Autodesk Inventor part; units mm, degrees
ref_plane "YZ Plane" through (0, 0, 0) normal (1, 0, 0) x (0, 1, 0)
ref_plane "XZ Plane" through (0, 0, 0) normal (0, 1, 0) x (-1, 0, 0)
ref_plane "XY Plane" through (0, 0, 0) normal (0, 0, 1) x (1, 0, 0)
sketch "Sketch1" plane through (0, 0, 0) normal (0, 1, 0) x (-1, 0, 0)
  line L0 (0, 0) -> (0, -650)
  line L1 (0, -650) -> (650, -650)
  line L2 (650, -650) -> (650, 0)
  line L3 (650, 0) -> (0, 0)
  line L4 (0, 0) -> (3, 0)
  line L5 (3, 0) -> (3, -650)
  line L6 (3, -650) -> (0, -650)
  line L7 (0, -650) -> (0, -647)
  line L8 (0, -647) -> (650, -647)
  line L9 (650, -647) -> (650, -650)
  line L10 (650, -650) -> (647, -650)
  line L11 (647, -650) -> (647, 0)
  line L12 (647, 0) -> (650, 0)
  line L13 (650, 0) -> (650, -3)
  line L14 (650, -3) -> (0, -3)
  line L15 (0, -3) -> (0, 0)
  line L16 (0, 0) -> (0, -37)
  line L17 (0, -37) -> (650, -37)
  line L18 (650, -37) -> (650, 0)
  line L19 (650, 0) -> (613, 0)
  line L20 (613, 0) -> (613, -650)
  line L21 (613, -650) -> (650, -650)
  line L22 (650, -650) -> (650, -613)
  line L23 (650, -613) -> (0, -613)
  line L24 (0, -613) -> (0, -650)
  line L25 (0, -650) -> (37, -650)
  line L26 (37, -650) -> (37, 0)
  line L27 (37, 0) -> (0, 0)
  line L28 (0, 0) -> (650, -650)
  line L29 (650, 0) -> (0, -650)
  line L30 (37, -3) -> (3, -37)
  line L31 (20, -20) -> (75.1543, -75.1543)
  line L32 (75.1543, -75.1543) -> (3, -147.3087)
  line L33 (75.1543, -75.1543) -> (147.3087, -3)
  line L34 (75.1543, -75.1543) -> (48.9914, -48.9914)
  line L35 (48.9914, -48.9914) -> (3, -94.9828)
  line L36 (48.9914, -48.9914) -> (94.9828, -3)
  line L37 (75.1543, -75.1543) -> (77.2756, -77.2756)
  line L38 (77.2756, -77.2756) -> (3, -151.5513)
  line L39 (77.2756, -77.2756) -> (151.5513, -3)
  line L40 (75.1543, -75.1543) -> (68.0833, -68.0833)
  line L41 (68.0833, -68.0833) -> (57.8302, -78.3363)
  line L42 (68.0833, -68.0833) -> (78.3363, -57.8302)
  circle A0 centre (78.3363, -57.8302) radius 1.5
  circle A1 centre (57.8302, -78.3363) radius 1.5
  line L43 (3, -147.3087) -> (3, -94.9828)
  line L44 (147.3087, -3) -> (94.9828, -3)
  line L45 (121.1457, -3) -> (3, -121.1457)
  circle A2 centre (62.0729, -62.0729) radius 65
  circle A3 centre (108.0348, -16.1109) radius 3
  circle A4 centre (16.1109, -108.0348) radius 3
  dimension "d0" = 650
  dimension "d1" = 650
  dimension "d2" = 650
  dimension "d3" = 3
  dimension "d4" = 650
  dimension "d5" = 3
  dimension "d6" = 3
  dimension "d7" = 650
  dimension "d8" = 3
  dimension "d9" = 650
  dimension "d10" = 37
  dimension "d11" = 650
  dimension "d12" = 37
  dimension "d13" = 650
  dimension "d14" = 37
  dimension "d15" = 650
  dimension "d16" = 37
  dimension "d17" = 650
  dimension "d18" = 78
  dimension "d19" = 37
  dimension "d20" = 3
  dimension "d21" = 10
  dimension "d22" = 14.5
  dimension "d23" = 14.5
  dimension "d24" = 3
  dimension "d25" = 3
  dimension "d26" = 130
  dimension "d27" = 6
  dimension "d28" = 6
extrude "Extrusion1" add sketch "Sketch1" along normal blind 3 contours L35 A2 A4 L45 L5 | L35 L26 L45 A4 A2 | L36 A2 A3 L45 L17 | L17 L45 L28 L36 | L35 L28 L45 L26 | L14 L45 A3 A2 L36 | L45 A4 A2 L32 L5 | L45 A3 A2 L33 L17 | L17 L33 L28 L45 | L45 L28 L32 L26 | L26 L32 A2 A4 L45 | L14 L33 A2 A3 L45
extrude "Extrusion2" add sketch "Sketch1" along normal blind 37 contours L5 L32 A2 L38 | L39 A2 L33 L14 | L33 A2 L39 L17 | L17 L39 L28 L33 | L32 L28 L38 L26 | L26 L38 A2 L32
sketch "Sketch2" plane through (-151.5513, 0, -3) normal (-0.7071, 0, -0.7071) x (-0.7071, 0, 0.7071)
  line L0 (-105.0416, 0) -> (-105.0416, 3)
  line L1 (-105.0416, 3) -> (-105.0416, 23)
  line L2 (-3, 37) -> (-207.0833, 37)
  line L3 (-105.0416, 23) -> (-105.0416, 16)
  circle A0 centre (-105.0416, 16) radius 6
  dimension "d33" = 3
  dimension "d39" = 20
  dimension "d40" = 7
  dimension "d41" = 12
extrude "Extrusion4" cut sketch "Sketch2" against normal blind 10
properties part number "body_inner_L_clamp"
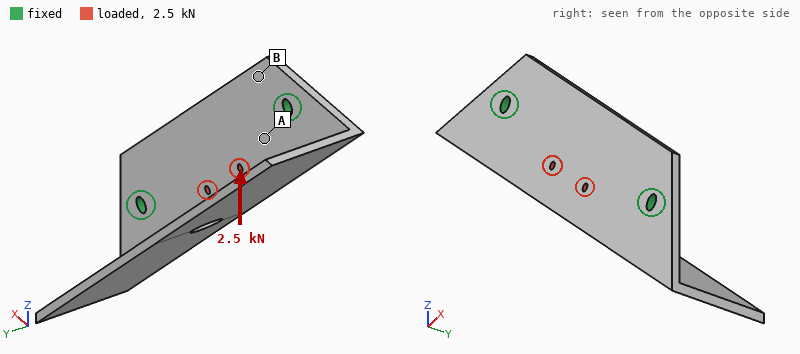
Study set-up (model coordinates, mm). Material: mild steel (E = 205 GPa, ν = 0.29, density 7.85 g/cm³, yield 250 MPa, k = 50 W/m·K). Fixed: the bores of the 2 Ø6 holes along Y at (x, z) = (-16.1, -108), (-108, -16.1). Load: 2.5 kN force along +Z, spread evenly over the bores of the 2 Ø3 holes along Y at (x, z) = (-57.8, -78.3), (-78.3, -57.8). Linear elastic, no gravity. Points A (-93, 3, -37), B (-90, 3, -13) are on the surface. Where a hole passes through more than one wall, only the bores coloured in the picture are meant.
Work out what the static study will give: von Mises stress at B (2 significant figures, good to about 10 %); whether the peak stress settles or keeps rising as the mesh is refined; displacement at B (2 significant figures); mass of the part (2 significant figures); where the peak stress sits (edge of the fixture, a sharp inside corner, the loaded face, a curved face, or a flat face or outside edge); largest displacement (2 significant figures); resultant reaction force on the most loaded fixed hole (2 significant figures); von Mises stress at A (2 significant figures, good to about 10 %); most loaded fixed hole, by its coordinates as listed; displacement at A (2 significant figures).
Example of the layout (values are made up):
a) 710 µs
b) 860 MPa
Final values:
a) 9.6 MPa
b) keeps rising
c) 7.0 µm
d) 320 g
e) edge of the fixture
f) 22 µm
g) 1.6 kN
h) 24 MPa
i) (-108, -16.1)
j) 10 µm
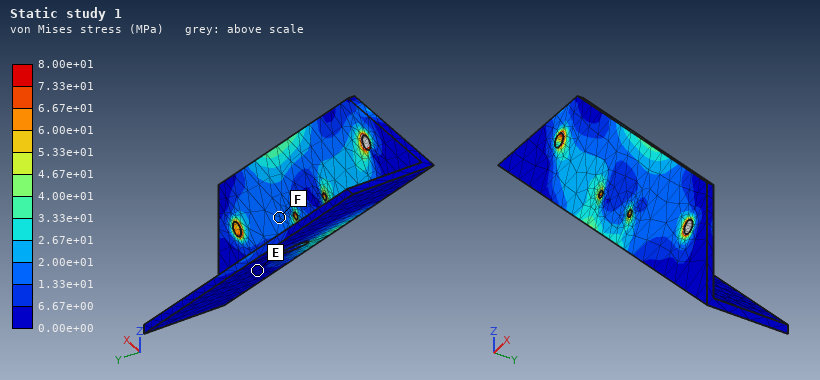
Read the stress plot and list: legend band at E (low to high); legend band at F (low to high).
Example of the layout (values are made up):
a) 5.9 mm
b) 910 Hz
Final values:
a) 0.00e+00 to 6.67e+00 MPa
b) 1.33e+01 to 2.00e+01 MPa
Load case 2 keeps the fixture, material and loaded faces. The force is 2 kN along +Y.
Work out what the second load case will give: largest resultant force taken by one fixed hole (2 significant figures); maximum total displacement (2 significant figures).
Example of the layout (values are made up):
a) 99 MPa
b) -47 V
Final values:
a) 1.1 kN
b) 0.27 mm
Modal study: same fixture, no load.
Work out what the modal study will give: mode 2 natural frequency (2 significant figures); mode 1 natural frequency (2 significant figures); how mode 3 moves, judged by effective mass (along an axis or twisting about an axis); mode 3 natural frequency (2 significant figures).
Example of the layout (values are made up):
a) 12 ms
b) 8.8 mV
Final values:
a) 1000 Hz
b) 770 Hz
c) along Y
d) 1400 Hz
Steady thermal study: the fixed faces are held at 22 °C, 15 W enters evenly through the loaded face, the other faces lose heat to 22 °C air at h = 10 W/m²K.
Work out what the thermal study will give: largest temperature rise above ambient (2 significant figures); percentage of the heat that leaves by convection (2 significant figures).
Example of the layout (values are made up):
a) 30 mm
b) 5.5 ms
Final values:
a) 53 K
b) 36 %
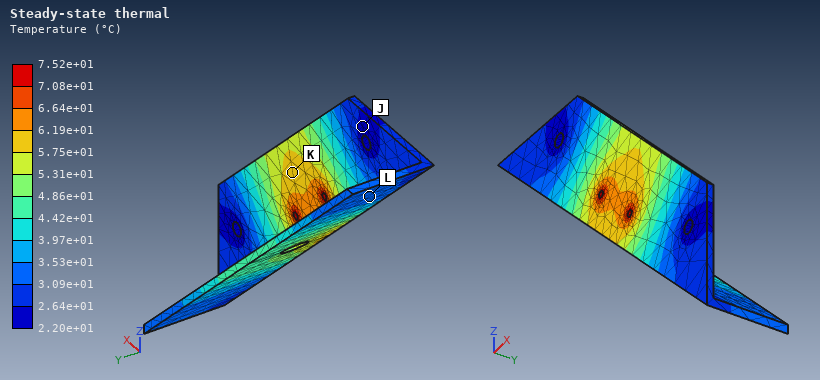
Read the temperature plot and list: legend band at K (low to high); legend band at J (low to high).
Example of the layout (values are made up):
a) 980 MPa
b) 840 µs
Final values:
a) 5.75e+01 to 6.19e+01 °C
b) 2.20e+01 to 2.64e+01 °C
